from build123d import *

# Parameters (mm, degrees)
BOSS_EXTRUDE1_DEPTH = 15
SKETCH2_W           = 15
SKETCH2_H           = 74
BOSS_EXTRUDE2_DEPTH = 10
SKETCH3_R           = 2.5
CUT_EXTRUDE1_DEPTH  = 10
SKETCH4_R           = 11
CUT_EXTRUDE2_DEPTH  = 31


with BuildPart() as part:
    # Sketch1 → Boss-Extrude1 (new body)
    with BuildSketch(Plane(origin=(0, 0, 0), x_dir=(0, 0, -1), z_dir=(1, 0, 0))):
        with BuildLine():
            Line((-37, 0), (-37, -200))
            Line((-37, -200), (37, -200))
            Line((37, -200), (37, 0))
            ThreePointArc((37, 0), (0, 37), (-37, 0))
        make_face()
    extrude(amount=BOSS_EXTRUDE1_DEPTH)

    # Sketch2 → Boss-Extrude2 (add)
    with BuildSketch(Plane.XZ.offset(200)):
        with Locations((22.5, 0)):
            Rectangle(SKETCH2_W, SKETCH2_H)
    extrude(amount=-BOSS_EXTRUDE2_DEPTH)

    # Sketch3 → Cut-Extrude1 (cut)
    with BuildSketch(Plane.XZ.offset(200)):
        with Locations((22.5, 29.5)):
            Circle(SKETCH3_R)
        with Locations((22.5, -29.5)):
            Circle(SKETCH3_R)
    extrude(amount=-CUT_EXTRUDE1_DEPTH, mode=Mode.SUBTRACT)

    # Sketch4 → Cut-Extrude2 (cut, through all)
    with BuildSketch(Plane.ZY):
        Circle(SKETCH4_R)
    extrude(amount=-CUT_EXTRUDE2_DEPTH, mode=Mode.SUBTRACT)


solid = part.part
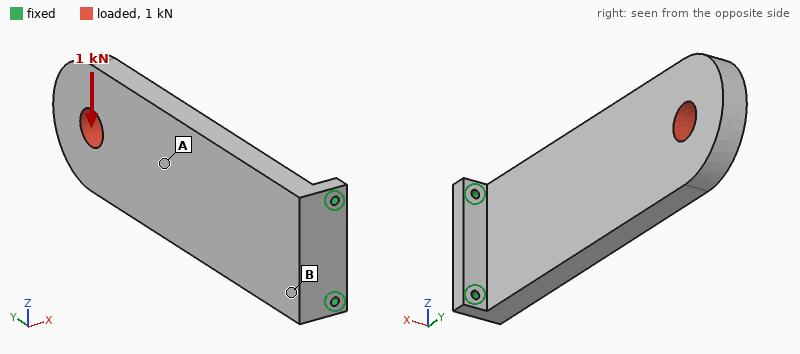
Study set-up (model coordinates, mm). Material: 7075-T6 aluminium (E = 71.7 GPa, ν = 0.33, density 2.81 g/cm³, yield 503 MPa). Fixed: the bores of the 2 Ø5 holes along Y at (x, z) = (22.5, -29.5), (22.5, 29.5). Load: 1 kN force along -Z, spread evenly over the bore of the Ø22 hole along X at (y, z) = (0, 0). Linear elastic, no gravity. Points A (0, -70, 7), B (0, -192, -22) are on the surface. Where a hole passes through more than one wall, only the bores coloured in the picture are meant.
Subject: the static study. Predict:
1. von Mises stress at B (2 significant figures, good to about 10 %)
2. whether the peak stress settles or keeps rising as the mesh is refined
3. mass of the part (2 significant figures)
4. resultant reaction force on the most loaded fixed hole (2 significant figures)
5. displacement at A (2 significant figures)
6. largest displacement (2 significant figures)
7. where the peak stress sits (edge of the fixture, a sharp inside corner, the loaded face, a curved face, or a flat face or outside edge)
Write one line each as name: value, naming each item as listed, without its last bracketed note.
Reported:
von Mises stress at B: 14 MPa
whether the peak stress settles or keeps rising as the mesh is refined: keeps rising
mass of the part: 730 g
resultant reaction force on the most loaded fixed hole: 3.3 kN
displacement at A: 0.10 mm
largest displacement: 0.23 mm
where the peak stress sits: edge of the fixture
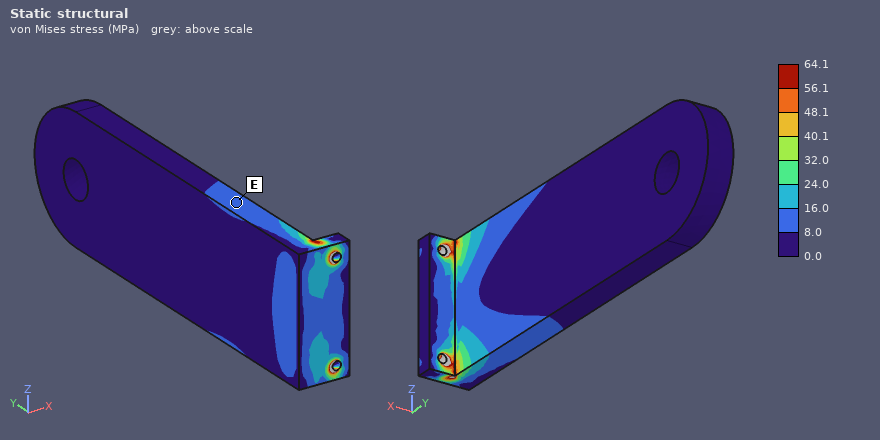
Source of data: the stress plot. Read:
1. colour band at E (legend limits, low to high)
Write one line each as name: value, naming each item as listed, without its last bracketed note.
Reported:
colour band at E: 8.0 to 16.0 MPa
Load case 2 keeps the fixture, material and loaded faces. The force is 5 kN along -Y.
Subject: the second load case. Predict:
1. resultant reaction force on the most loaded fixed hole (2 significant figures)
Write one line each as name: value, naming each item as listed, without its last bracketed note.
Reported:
resultant reaction force on the most loaded fixed hole: 2.5 kN
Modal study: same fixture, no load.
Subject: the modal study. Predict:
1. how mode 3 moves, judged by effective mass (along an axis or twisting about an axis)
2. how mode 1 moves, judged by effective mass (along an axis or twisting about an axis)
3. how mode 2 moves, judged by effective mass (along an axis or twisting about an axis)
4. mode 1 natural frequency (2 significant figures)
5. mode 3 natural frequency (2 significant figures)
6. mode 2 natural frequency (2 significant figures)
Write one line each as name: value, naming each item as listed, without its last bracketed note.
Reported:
how mode 3 moves, judged by effective mass: along X
how mode 1 moves, judged by effective mass: along X
how mode 2 moves, judged by effective mass: along Z
mode 1 natural frequency: 170 Hz
mode 3 natural frequency: 1200 Hz
mode 2 natural frequency: 690 Hz
